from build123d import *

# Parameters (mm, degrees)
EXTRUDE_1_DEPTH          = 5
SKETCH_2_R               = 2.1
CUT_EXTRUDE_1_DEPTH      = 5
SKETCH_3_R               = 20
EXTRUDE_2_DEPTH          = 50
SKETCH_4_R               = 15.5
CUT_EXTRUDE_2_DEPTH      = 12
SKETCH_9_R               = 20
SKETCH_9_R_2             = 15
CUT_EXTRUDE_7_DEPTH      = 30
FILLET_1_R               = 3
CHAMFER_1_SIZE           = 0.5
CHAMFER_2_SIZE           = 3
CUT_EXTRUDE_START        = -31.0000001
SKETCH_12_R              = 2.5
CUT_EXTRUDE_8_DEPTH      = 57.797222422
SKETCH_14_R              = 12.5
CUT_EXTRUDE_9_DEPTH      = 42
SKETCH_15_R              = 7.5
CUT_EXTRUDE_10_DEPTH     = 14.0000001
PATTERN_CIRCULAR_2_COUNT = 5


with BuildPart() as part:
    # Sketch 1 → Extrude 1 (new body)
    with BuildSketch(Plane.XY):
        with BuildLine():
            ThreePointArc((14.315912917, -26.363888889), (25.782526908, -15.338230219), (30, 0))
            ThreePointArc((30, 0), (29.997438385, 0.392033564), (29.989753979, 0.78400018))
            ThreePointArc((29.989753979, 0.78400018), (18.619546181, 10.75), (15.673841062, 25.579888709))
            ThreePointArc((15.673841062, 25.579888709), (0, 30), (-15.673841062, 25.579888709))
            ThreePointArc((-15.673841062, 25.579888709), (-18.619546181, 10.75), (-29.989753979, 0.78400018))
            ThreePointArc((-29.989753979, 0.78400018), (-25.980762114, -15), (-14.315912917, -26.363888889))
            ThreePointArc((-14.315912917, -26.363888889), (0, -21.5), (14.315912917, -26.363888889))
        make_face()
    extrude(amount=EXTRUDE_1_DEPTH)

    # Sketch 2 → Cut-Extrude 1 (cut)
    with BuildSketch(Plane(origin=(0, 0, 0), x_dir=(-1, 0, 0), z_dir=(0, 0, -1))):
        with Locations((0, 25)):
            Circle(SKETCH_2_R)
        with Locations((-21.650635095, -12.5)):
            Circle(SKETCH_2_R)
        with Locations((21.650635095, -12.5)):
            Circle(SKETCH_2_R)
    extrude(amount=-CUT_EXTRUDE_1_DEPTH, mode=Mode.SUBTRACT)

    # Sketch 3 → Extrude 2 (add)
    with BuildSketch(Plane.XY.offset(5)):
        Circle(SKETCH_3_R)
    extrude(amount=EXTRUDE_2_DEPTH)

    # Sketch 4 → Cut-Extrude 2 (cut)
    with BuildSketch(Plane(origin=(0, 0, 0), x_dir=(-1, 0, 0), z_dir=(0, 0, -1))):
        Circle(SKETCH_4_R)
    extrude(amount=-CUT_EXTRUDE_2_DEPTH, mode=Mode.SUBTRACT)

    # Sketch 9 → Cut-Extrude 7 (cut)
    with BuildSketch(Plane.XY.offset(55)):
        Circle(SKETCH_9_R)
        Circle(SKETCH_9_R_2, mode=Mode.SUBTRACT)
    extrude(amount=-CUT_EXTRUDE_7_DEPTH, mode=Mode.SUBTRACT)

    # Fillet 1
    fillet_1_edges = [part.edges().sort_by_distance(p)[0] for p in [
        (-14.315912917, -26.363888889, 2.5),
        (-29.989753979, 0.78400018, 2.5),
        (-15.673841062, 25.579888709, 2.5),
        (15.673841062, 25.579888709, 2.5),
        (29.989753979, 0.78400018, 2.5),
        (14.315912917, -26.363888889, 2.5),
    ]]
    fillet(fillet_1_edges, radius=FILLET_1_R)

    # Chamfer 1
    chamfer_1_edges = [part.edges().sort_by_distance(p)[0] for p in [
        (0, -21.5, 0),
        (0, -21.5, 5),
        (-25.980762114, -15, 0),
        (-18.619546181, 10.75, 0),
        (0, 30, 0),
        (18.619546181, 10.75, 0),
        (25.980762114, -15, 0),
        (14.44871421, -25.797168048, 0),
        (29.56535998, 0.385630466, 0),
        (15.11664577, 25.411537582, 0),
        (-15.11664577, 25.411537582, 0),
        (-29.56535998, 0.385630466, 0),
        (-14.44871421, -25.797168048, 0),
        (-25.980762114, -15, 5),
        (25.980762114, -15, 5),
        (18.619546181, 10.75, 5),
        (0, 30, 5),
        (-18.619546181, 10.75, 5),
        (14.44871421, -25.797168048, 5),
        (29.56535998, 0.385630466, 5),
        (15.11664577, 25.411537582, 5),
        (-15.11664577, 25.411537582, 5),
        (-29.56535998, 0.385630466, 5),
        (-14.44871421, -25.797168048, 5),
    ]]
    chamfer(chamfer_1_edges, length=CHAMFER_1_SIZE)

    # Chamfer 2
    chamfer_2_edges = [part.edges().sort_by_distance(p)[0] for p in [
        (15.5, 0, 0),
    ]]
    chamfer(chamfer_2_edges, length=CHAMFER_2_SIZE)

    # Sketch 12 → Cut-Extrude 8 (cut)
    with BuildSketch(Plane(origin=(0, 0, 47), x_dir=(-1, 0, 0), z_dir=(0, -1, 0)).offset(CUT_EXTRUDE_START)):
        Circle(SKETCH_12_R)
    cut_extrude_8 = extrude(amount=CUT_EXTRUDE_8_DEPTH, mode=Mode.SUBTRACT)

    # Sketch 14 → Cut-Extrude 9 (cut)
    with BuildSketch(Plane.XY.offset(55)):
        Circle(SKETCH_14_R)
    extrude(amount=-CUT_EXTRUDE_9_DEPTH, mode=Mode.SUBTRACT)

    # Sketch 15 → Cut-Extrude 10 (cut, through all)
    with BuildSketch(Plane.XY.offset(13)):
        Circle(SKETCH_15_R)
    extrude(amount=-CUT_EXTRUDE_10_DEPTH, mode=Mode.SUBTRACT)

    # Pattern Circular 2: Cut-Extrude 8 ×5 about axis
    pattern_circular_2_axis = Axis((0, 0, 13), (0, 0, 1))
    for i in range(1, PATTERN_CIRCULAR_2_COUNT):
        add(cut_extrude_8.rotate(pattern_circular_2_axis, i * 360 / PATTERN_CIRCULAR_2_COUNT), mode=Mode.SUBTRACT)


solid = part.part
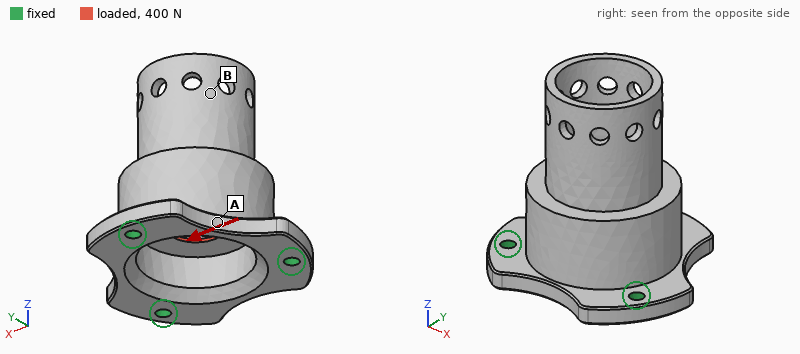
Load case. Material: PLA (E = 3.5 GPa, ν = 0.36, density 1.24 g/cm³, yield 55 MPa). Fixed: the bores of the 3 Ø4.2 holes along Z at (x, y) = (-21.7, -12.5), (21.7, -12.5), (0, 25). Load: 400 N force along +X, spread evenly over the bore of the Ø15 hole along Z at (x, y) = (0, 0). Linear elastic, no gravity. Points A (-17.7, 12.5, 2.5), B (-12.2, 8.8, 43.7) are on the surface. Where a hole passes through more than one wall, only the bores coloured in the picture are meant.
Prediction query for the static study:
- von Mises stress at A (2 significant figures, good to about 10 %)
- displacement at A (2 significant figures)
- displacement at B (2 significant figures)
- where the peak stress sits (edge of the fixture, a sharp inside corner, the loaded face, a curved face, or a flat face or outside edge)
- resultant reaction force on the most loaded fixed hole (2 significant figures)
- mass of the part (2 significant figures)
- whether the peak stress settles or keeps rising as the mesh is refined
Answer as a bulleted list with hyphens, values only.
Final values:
- 2.3 MPa
- 21 µm
- 49 µm
- a sharp inside corner
- 160 N
- 33 g
- keeps rising
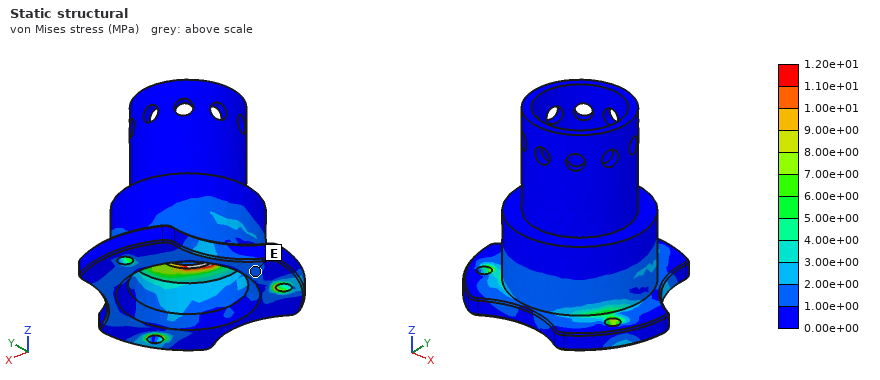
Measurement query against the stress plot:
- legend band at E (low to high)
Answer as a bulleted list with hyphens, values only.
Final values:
- 1.00e+00 to 2.00e+00 MPa
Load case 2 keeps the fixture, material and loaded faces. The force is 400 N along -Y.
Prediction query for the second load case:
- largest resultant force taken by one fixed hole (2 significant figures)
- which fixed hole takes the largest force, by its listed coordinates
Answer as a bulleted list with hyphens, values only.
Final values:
- 170 N
- (0, 25)
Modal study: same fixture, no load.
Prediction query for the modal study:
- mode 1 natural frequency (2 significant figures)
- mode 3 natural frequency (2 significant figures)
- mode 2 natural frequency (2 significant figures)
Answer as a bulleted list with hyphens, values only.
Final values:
- 2100 Hz
- 3600 Hz
- 2100 Hz
